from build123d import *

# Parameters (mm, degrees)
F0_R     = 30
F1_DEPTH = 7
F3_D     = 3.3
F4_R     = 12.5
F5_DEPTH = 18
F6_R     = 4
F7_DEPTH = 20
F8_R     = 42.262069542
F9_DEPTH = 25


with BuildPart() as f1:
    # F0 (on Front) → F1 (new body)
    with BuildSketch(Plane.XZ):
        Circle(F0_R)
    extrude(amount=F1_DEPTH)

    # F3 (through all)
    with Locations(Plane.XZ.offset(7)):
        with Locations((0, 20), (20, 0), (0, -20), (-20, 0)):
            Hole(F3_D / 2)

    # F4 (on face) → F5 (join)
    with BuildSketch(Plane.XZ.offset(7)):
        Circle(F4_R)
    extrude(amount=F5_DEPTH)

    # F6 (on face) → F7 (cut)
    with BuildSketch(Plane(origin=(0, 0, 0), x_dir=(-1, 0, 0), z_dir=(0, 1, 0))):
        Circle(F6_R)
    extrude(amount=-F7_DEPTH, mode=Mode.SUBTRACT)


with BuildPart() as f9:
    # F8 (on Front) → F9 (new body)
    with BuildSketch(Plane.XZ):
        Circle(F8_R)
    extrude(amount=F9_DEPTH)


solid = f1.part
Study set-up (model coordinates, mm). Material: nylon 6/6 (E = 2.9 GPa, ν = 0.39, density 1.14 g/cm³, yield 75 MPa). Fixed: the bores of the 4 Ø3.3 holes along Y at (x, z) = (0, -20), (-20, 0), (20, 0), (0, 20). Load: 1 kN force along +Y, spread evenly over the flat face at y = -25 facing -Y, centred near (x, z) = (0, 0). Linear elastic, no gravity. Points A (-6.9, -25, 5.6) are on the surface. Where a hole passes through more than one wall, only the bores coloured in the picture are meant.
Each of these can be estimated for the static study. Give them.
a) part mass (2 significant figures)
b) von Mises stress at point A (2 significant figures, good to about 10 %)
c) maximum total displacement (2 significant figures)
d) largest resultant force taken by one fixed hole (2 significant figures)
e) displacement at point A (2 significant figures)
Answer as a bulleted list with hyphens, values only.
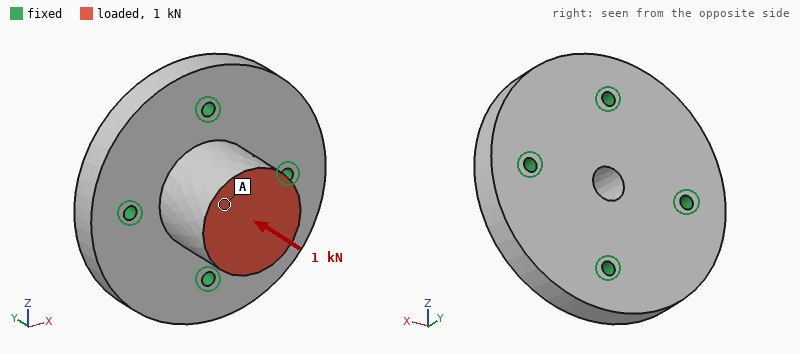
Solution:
- 31 g
- 2.1 MPa
- 57 µm
- 260 N
- 55 µm
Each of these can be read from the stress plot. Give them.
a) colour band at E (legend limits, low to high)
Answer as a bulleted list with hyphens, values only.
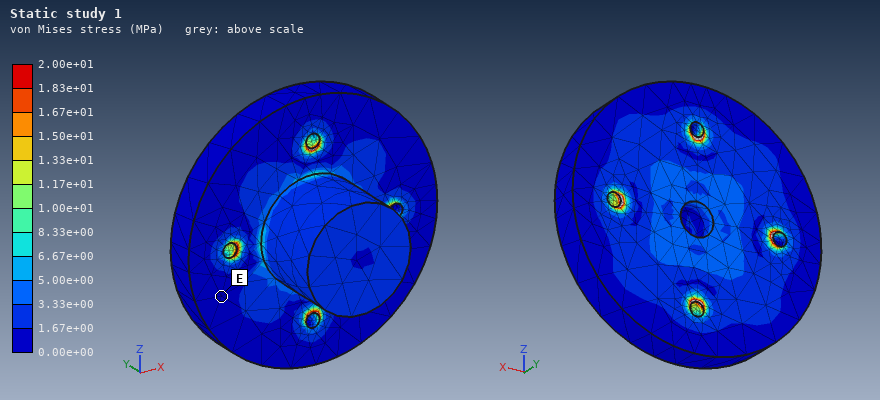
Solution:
- 0.00e+00 to 1.67e+00 MPa
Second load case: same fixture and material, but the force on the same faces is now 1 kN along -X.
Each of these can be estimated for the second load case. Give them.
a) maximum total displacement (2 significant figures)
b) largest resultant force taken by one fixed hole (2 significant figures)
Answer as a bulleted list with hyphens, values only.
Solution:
- 0.24 mm
- 650 N
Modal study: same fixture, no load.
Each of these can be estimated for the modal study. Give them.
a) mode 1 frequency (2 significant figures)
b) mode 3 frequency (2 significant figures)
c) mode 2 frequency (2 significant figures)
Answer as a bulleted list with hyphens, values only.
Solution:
- 5000 Hz
- 5800 Hz
- 5000 Hz
